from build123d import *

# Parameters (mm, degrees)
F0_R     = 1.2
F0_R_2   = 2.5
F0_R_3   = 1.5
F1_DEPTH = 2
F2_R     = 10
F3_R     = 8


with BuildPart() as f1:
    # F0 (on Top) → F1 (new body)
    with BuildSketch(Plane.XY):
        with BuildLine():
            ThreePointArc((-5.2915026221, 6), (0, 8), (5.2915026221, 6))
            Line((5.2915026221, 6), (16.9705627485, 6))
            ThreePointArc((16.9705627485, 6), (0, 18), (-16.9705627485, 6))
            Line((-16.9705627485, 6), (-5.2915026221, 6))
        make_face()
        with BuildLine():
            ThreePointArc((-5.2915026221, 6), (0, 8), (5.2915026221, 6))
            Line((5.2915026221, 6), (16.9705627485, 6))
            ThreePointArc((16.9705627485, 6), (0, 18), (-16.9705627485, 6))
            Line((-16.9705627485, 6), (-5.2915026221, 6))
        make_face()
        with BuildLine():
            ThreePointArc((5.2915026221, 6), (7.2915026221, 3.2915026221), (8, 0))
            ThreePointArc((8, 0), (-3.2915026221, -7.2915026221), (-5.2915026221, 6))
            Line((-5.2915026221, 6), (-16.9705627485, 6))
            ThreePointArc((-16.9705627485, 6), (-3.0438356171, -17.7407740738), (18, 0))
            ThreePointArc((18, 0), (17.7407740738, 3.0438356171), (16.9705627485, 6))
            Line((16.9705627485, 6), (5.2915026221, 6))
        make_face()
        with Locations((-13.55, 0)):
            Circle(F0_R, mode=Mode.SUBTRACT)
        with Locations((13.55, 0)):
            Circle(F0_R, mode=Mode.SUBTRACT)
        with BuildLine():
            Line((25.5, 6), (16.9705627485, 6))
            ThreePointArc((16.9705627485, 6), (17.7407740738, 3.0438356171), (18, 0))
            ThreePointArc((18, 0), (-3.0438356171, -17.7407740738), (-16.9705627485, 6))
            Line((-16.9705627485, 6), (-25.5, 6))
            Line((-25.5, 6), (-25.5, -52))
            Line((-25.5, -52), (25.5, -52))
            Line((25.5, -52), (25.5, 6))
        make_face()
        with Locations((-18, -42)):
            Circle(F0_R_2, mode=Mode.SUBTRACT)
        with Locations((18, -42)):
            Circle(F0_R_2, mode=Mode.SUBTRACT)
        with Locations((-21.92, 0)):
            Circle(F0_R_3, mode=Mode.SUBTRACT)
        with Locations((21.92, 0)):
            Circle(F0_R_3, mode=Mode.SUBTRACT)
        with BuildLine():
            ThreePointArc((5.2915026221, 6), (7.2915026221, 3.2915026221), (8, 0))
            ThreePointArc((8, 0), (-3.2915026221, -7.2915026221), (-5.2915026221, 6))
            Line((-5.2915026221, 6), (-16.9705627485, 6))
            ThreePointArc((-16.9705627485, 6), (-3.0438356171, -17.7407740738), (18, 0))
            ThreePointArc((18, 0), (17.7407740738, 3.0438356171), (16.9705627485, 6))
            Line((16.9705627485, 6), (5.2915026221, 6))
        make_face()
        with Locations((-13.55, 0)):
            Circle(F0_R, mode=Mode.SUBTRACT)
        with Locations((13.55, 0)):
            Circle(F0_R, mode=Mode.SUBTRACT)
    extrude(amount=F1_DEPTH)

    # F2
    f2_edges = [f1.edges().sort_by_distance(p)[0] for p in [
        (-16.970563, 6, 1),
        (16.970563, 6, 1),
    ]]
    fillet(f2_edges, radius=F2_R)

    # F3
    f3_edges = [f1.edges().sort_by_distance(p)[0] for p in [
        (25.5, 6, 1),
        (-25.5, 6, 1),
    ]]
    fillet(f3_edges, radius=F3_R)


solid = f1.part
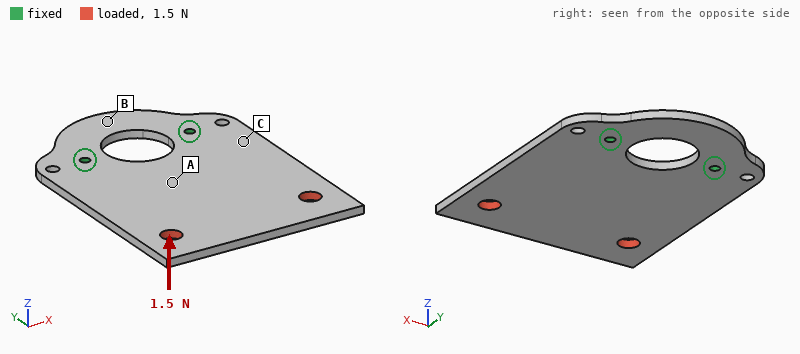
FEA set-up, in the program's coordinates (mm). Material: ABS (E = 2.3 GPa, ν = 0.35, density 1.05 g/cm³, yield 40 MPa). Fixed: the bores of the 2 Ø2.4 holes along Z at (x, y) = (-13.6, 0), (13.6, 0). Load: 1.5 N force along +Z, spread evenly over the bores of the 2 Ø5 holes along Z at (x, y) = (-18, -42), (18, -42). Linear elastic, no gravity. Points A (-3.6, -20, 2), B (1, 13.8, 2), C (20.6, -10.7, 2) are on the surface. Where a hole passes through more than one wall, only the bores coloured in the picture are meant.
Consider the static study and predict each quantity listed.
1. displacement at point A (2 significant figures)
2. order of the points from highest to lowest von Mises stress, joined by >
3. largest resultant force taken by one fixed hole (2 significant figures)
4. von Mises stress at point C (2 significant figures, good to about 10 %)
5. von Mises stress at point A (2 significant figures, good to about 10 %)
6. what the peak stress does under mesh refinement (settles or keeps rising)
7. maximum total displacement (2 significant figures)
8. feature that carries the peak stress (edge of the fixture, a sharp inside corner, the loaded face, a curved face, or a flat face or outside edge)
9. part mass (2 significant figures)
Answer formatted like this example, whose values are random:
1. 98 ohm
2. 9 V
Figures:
1. 0.20 mm
2. C > A > B
3. 0.75 N
4. 1.5 MPa
5. 0.80 MPa
6. keeps rising
7. 0.80 mm
8. edge of the fixture
9. 6.3 g
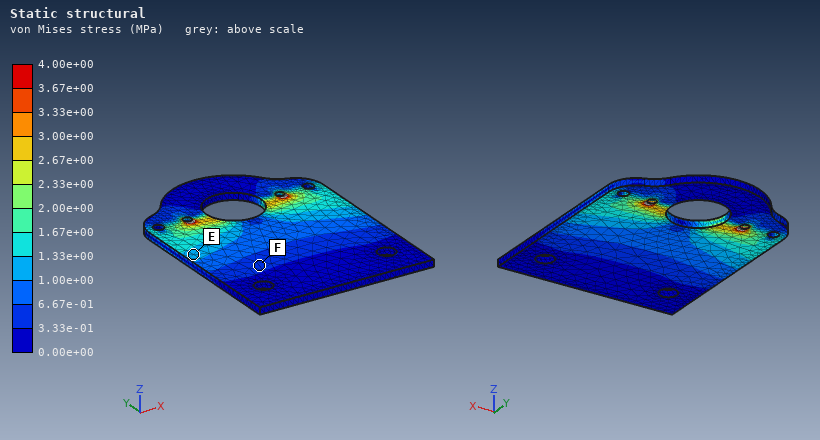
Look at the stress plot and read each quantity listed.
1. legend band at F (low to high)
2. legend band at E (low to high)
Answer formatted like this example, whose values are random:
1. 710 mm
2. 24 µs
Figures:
1. 3.33e-01 to 6.67e-01 MPa
2. 1.00e+00 to 1.33e+00 MPa
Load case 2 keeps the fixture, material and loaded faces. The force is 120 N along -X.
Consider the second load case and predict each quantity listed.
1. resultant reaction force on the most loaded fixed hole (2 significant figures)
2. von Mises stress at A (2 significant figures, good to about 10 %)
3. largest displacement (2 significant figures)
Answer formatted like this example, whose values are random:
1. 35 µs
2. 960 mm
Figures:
1. 180 N
2. 4.6 MPa
3. 0.31 mm
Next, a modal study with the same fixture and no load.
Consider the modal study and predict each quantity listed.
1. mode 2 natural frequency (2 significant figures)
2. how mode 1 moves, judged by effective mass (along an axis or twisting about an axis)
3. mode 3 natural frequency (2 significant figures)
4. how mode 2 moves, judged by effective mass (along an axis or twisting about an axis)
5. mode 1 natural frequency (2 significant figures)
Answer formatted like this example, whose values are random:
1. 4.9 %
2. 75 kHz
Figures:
1. 420 Hz
2. along Z
3. 1000 Hz
4. twisting about Y
5. 160 Hz
